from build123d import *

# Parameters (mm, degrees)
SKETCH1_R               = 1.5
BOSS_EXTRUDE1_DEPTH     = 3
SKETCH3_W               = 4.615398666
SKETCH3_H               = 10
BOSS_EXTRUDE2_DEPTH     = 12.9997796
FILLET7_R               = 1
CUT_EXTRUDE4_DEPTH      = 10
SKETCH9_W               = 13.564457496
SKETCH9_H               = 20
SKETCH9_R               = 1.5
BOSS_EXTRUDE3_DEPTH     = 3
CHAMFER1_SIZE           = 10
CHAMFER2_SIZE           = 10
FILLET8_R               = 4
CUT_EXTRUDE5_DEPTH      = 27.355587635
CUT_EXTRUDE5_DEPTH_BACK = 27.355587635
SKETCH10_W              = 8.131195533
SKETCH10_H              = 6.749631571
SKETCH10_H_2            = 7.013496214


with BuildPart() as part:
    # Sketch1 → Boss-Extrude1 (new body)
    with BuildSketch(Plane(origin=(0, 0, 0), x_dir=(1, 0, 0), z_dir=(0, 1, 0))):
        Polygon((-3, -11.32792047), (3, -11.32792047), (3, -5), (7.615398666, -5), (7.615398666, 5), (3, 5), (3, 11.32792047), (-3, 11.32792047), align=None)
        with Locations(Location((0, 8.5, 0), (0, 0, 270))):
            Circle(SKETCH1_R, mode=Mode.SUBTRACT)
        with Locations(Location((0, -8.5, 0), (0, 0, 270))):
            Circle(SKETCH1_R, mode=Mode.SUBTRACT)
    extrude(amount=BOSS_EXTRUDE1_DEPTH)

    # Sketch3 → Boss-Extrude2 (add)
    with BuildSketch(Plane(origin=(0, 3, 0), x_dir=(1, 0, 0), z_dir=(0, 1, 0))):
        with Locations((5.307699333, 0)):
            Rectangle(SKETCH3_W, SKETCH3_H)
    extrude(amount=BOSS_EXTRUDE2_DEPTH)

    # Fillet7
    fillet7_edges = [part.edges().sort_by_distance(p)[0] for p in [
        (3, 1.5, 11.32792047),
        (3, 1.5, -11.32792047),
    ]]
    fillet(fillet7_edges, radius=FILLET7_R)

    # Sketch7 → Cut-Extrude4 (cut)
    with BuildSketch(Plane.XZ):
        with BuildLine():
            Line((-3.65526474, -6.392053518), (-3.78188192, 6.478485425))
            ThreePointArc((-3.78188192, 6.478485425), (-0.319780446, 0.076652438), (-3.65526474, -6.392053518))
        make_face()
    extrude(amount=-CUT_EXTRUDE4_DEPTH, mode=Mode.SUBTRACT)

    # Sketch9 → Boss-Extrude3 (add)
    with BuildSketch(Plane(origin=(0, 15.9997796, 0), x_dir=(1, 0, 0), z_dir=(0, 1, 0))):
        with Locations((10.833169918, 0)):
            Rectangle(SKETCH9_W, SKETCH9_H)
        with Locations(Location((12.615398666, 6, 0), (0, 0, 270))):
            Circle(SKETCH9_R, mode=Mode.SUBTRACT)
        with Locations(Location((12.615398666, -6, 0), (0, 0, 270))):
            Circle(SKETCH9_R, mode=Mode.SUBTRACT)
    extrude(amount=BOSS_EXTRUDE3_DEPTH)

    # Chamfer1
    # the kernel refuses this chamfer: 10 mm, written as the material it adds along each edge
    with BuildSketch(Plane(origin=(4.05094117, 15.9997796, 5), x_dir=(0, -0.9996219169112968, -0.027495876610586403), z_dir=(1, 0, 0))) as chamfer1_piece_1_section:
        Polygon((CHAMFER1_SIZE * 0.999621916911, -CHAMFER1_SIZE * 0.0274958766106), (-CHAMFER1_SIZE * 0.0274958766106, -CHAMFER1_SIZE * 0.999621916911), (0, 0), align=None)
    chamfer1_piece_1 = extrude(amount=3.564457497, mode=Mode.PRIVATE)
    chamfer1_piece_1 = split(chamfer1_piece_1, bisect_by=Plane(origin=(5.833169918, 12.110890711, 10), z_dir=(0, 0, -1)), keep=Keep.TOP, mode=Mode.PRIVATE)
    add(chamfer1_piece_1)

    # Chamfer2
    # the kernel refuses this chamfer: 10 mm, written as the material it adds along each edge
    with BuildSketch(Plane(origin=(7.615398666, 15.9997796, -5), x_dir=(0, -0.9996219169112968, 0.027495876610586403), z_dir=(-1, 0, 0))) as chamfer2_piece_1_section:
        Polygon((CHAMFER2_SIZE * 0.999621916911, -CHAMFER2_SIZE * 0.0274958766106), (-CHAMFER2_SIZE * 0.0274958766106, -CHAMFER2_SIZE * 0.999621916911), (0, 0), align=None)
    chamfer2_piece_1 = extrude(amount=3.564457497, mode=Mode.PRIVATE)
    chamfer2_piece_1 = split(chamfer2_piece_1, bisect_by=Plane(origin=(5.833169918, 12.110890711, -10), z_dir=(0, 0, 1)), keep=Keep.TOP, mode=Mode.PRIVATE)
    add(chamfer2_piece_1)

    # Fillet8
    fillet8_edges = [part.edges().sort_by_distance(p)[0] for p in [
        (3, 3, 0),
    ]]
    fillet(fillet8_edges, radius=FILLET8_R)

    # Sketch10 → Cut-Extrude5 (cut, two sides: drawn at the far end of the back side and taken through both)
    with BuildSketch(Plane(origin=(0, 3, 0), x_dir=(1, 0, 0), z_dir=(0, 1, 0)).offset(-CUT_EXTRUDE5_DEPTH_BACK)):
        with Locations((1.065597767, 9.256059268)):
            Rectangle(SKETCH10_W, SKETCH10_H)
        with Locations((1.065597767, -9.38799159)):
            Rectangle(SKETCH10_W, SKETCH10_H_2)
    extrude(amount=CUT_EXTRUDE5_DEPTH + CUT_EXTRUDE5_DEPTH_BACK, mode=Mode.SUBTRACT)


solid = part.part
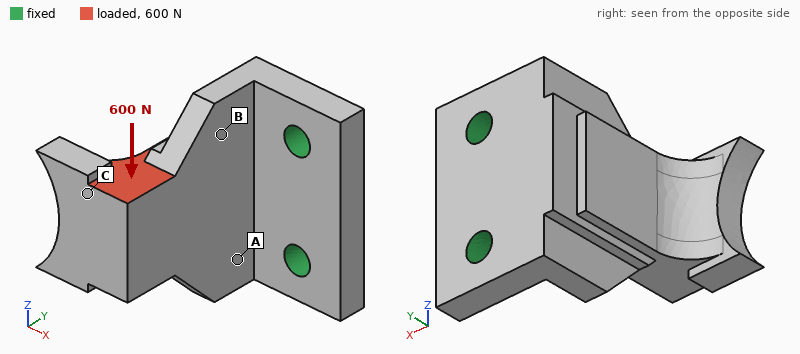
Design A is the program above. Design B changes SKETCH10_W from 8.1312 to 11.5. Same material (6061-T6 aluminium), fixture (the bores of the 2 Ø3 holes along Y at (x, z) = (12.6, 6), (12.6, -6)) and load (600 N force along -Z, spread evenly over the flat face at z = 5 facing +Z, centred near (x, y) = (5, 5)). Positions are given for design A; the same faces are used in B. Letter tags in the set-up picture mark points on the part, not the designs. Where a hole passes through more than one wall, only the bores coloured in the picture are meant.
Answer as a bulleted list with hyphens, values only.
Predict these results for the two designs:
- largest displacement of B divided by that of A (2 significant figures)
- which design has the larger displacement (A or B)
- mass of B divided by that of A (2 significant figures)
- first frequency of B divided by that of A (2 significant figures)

- 1.1
- B
- 0.93
- 0.92
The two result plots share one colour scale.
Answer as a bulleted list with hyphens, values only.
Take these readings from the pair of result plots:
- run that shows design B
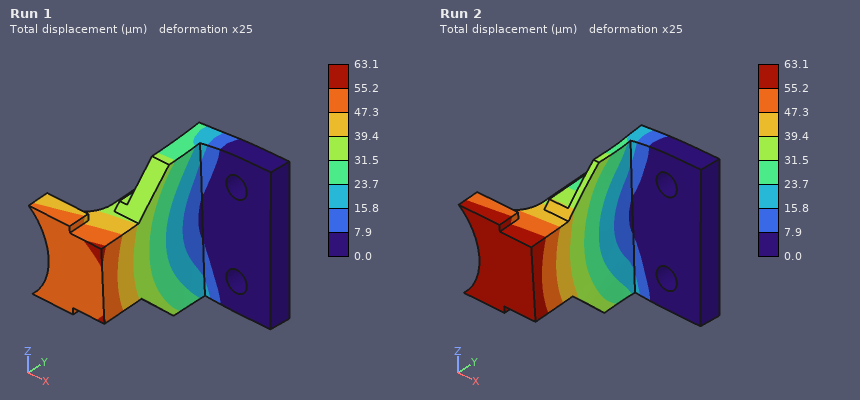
- Run 2
